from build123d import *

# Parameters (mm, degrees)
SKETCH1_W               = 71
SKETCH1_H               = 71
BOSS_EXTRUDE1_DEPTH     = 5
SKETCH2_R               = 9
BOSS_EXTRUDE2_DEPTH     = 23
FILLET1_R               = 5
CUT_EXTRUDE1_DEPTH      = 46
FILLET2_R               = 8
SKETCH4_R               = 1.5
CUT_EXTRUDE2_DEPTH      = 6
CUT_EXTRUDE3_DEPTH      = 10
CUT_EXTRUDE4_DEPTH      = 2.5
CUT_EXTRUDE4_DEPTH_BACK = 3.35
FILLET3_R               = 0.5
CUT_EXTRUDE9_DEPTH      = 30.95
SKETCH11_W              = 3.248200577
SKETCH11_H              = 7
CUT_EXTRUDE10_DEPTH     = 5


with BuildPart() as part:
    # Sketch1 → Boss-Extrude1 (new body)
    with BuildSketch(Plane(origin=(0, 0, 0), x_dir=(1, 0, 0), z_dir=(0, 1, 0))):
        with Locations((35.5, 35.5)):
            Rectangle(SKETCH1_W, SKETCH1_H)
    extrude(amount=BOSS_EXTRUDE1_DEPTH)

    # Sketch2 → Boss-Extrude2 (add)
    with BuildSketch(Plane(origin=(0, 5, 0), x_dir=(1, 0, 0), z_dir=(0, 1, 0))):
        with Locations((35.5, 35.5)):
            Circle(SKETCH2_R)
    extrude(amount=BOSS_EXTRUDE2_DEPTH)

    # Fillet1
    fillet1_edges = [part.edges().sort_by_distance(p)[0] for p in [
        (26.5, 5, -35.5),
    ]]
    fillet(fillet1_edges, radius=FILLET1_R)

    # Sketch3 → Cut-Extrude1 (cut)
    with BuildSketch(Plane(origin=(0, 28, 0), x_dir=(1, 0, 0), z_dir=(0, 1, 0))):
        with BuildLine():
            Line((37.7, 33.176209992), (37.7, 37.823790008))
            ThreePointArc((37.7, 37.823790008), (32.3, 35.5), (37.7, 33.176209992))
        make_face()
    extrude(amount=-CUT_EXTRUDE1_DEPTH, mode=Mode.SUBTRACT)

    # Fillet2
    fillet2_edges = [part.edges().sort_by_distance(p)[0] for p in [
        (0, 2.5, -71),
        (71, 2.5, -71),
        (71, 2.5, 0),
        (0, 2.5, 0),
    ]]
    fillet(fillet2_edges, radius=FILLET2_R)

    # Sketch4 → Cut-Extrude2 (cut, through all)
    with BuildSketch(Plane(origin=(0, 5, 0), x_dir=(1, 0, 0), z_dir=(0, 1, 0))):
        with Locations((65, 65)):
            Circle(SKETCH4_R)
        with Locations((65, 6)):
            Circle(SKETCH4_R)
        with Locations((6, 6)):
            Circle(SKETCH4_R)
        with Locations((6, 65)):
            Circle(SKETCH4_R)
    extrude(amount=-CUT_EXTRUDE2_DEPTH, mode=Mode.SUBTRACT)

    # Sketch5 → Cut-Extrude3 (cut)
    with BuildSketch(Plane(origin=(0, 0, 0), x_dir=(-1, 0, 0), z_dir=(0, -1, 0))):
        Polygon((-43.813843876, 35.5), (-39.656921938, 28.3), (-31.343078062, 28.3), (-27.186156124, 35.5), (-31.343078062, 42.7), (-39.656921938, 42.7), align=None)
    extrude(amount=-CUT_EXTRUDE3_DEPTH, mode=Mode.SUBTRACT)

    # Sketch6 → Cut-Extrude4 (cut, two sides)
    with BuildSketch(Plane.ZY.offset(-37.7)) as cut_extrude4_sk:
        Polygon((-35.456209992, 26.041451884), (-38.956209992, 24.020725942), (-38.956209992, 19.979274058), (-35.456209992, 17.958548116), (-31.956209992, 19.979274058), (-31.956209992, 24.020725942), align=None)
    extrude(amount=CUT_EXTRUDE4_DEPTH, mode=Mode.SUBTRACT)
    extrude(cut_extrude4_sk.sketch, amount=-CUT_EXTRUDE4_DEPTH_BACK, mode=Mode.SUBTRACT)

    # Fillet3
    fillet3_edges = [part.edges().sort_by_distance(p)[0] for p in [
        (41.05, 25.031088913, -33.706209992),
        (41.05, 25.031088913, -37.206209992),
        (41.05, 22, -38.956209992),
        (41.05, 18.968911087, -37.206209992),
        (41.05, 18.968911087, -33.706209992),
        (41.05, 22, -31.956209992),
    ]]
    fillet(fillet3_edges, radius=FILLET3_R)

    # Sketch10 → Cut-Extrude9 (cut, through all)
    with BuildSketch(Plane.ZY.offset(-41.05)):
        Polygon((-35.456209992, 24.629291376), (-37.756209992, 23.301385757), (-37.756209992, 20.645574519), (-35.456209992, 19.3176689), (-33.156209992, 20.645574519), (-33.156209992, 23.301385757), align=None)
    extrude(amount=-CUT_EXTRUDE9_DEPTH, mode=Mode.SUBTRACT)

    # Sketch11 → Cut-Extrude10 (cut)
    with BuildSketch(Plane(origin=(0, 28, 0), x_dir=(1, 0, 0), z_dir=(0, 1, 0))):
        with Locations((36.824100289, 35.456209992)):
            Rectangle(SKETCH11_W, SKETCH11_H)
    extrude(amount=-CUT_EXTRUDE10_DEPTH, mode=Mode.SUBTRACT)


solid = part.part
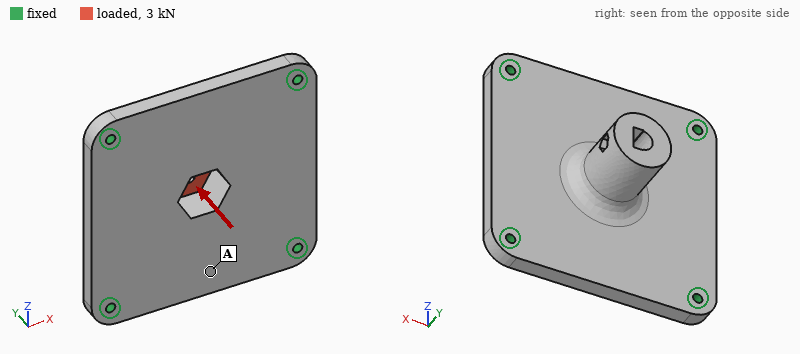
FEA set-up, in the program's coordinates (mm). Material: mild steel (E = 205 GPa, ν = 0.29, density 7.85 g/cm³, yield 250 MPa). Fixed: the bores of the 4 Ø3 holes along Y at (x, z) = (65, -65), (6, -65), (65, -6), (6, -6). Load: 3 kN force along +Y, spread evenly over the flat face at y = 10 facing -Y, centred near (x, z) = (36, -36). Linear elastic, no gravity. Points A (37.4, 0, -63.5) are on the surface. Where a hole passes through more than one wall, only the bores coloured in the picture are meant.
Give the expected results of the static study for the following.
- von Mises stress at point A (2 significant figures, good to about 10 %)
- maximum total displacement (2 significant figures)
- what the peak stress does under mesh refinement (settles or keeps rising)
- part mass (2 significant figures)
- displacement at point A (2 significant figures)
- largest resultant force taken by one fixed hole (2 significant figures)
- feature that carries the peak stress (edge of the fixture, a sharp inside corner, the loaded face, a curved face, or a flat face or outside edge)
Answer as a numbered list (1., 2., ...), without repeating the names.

1. 49 MPa
2. 53 µm
3. keeps rising
4. 220 g
5. 25 µm
6. 800 N
7. edge of the fixture
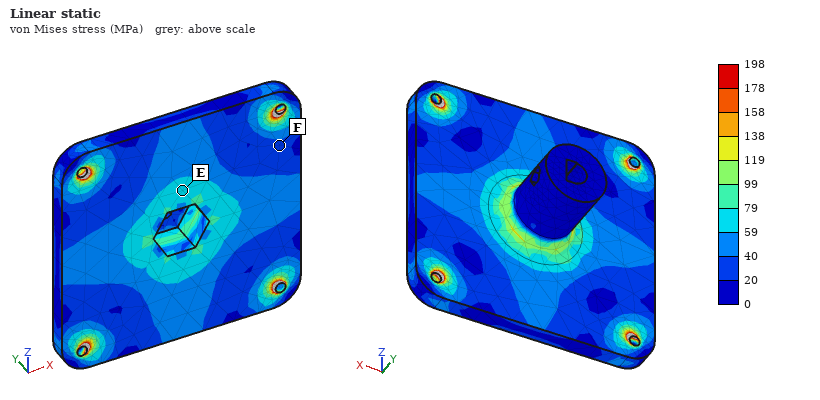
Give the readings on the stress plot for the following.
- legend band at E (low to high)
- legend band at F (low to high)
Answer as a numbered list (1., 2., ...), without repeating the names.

1. 59 to 79 MPa
2. 20 to 40 MPa
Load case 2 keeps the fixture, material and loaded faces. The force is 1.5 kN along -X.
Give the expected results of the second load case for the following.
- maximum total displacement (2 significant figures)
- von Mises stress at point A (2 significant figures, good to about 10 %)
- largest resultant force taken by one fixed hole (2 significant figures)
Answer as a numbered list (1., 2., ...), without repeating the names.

1. 11 µm
2. 4.6 MPa
3. 430 N
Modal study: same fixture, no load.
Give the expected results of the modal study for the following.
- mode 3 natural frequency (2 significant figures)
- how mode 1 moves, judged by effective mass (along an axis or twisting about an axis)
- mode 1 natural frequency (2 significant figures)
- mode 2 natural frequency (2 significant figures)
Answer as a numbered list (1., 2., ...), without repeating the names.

1. 6000 Hz
2. along Y
3. 4000 Hz
4. 6000 Hz
